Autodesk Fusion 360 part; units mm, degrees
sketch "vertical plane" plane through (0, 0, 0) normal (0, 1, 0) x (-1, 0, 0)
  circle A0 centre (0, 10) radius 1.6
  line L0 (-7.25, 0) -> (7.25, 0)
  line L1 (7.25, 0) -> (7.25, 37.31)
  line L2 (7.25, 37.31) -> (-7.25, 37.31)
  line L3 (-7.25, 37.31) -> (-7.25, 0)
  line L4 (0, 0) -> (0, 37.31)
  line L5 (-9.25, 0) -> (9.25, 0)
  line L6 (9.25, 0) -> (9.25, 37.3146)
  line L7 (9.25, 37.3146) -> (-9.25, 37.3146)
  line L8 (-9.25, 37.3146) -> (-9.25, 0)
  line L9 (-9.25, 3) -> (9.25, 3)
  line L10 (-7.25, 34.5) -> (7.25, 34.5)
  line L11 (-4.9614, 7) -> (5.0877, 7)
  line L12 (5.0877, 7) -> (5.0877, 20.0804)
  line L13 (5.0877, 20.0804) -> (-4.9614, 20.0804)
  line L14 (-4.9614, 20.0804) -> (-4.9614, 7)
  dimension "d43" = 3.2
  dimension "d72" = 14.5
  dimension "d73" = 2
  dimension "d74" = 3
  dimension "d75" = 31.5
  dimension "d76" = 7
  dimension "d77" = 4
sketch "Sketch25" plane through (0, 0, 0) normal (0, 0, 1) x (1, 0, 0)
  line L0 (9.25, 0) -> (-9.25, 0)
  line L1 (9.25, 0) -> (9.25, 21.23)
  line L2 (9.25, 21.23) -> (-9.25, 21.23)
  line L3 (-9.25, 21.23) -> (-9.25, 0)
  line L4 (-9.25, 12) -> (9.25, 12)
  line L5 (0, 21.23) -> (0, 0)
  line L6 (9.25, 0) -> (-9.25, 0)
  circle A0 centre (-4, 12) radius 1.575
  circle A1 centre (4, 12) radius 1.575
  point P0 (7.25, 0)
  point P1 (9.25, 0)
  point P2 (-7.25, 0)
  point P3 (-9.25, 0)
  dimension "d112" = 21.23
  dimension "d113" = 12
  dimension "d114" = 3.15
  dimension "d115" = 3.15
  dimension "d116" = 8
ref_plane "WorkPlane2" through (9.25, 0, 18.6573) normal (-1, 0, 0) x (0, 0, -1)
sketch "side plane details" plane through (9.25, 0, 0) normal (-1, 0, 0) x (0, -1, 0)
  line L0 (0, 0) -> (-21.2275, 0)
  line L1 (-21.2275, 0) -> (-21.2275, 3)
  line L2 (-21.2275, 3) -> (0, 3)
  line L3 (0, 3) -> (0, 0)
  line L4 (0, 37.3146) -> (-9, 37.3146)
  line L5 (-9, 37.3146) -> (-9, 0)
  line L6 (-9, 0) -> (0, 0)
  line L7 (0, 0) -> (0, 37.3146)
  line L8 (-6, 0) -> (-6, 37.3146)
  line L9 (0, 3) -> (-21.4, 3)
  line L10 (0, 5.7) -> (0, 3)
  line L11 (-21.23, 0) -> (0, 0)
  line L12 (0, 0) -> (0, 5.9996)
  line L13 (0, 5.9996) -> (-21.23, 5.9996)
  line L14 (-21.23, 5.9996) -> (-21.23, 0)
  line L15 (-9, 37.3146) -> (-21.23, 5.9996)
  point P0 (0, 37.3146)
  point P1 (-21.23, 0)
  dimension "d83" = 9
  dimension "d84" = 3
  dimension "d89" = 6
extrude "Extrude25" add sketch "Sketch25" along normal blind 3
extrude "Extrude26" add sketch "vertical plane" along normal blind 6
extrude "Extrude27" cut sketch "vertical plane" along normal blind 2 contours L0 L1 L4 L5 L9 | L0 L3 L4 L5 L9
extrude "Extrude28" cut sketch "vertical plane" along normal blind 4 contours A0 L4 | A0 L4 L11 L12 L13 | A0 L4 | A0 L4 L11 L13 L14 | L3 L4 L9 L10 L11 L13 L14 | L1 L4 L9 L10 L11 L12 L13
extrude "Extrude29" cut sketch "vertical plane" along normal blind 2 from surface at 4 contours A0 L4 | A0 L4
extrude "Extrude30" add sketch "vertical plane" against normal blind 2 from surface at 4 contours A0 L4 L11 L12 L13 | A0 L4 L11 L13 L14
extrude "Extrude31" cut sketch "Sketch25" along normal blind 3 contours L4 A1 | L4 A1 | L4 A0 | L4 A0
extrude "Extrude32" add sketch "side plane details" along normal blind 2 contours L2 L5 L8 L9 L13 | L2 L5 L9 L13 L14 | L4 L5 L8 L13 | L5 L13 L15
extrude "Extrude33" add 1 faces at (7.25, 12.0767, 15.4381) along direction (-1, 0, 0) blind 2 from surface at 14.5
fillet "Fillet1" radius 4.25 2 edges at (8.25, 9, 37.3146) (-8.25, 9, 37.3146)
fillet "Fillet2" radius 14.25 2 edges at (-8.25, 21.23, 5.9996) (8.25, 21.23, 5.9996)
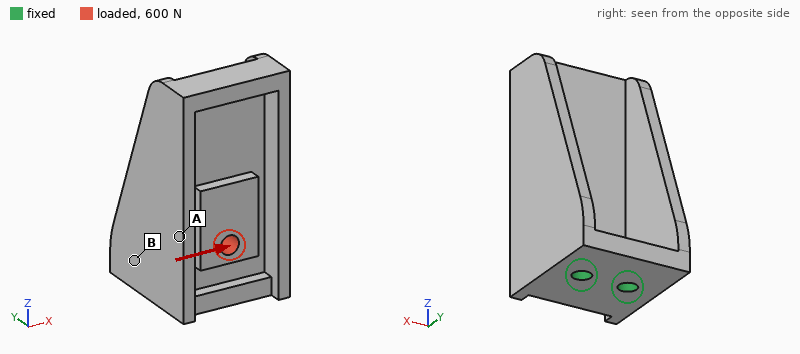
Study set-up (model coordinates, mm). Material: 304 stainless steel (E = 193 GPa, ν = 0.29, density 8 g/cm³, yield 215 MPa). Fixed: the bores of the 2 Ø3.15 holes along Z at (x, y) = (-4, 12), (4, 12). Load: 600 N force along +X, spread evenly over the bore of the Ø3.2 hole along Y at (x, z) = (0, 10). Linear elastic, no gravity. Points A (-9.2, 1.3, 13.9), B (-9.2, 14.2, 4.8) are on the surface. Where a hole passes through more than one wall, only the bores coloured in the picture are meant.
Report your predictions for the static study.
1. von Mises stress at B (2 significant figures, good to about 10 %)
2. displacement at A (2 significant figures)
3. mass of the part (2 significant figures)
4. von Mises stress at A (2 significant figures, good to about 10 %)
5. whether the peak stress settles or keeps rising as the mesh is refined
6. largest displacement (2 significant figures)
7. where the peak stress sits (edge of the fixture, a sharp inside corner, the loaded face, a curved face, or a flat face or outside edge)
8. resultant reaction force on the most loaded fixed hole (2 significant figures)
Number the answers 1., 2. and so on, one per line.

1. 20 MPa
2. 9.7 µm
3. 37 g
4. 9.4 MPa
5. keeps rising
6. 23 µm
7. edge of the fixture
8. 640 N
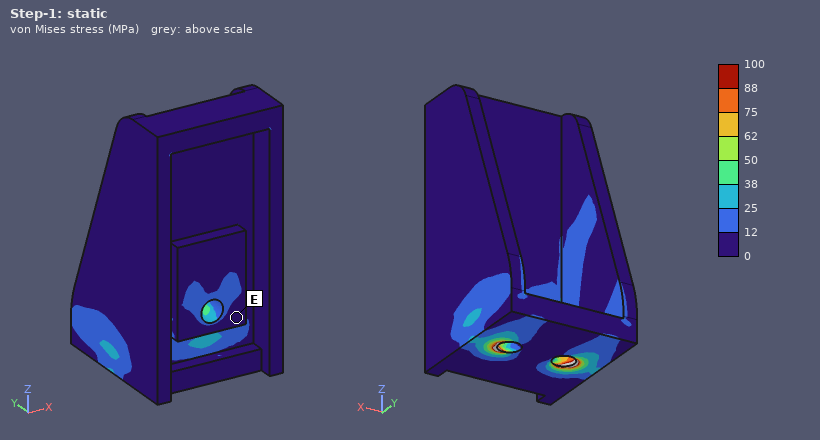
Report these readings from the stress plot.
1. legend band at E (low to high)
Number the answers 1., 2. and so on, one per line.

1. 0 to 12 MPa
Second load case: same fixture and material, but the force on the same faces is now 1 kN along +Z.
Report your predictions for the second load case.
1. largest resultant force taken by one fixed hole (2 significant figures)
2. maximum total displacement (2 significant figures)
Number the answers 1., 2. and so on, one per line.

1. 500 N
2. 44 µm
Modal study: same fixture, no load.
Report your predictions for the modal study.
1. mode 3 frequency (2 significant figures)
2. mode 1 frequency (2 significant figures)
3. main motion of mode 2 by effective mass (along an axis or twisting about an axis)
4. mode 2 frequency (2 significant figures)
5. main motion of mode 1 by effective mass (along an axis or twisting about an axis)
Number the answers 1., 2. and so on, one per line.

1. 8700 Hz
2. 3400 Hz
3. along X
4. 3800 Hz
5. along Y
